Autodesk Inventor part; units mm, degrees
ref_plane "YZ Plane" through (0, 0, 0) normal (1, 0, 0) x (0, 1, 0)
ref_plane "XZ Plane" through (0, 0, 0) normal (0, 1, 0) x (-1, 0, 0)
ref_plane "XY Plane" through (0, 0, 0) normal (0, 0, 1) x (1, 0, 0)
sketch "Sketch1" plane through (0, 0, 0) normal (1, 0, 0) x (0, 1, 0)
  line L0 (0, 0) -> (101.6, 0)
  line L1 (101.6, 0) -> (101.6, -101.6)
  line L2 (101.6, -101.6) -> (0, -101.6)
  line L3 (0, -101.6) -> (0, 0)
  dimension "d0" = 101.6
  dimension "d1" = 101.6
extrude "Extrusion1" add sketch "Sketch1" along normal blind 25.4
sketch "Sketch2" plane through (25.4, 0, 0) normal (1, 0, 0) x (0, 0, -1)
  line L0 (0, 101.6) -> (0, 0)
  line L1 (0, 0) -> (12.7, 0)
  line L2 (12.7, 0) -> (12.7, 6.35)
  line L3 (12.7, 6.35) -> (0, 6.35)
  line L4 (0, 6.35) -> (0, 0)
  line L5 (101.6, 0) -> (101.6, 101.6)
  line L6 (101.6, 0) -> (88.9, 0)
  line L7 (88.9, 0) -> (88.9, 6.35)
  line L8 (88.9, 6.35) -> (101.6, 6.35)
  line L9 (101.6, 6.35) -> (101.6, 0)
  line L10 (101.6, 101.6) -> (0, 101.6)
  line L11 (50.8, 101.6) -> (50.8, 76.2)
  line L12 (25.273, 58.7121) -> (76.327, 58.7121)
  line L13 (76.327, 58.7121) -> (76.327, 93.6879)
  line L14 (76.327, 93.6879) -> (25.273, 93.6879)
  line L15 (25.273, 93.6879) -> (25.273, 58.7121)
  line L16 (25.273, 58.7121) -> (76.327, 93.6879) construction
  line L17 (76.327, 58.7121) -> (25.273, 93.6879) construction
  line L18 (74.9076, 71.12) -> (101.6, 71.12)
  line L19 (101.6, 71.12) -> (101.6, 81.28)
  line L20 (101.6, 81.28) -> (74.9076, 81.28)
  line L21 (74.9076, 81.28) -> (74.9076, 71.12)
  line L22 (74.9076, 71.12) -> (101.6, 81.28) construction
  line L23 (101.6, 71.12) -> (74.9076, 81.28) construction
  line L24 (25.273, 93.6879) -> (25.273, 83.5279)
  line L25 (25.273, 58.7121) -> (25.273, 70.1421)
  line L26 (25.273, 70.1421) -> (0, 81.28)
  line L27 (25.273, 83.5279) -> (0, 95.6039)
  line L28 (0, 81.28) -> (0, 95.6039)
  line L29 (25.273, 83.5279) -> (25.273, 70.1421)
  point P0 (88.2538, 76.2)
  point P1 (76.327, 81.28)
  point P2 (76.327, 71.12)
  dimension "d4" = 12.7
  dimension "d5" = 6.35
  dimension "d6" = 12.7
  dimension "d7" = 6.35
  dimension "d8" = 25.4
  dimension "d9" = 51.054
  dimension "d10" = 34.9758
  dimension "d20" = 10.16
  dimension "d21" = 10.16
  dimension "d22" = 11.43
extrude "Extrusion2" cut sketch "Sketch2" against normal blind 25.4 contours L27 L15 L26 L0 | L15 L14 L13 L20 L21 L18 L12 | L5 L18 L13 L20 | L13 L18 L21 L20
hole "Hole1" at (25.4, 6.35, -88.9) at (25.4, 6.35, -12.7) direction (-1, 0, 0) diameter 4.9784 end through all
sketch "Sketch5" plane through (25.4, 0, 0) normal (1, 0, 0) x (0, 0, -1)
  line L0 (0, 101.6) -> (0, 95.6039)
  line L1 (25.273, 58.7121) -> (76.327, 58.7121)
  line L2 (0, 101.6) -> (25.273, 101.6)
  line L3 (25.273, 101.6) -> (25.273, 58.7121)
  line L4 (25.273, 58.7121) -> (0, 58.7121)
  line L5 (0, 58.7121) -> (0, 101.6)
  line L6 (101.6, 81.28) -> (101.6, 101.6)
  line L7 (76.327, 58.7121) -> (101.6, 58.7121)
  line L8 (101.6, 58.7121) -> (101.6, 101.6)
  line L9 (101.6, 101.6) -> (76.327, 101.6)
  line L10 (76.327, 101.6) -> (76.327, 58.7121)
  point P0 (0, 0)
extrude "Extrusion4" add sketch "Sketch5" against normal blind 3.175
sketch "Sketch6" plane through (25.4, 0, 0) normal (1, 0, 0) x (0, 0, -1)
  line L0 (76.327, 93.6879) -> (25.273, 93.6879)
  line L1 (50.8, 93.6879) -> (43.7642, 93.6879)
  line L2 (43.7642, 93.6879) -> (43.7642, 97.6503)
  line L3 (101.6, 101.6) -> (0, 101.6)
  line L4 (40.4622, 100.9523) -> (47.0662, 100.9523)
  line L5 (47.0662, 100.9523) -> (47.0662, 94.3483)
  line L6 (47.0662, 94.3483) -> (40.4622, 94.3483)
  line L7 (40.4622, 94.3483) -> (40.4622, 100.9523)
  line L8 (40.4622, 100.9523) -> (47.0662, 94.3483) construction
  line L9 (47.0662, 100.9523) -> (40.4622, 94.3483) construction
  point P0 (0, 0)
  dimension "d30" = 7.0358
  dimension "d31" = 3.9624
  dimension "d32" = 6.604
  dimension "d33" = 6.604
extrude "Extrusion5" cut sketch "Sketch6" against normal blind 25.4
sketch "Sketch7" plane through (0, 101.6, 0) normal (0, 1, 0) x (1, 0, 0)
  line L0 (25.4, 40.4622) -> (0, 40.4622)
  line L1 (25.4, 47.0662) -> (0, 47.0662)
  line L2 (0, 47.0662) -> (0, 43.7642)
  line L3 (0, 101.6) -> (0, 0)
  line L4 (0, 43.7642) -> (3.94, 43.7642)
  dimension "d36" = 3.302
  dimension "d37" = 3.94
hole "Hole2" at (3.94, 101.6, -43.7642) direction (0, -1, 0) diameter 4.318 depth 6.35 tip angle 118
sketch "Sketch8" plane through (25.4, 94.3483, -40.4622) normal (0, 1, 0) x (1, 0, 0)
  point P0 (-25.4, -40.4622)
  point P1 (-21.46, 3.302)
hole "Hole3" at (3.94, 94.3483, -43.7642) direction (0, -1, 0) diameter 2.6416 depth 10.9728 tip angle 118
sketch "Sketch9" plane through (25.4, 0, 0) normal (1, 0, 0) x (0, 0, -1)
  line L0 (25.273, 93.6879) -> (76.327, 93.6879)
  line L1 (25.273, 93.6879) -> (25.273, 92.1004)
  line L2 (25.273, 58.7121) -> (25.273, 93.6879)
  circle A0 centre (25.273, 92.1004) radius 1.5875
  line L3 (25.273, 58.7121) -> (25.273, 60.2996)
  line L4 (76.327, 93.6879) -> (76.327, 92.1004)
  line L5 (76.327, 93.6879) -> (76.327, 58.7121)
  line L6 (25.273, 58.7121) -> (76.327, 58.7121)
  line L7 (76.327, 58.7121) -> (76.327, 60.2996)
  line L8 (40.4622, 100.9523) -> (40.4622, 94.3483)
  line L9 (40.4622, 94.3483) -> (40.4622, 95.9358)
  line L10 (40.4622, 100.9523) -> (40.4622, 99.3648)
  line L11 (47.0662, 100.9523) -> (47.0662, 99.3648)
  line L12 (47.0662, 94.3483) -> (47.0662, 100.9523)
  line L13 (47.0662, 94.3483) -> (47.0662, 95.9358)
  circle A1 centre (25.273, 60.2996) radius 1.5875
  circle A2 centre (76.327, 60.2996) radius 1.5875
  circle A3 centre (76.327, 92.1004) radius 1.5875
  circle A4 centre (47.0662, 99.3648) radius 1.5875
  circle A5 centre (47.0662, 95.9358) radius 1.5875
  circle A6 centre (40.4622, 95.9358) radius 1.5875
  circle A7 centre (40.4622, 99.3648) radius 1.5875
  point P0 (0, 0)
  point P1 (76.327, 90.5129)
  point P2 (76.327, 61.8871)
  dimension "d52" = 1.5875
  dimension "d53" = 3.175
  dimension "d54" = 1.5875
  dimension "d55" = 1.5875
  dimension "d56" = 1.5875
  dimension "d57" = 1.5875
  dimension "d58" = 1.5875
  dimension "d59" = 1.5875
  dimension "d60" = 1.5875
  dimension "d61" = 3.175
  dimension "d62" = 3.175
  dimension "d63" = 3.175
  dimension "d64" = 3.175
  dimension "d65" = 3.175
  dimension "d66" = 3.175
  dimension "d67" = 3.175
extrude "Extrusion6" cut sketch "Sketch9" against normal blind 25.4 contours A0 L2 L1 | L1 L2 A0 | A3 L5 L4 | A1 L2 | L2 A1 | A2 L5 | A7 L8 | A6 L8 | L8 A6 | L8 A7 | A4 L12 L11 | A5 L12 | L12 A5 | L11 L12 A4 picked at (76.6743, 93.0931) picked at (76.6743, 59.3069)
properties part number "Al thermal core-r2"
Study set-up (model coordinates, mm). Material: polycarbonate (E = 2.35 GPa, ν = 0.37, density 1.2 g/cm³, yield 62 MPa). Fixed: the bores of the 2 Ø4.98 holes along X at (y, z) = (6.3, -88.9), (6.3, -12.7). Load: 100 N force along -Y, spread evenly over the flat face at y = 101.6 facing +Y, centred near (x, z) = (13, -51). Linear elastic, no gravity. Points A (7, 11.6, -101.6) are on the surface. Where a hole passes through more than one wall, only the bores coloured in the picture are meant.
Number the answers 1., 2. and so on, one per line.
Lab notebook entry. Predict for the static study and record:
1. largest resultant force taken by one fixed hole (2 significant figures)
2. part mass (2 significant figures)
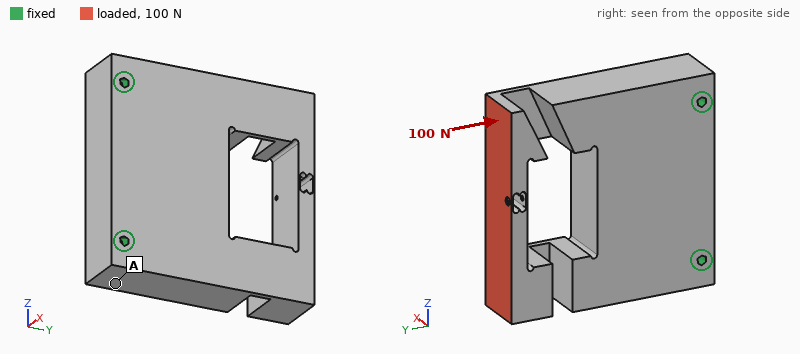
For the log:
1. 50 N
2. 240 g
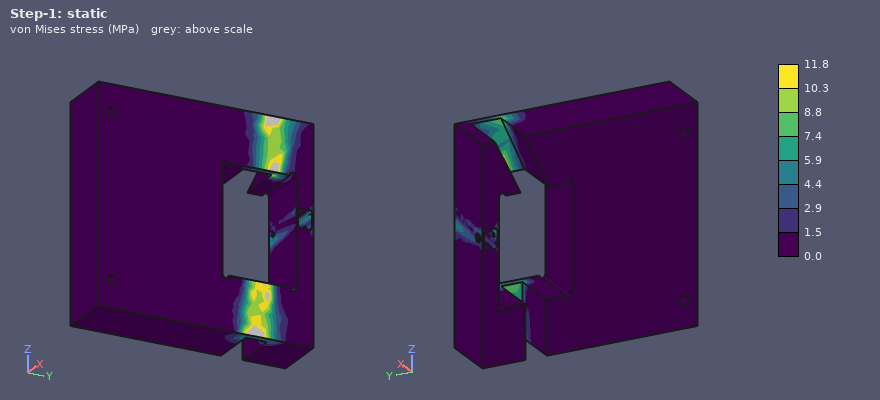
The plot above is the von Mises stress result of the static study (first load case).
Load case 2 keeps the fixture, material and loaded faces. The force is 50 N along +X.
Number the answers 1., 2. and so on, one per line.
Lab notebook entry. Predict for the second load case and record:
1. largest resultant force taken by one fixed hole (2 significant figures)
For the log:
1. 25 N
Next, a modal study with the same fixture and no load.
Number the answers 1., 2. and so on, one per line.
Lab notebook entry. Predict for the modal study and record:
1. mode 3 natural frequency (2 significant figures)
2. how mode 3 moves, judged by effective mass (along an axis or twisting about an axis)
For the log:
1. 700 Hz
2. along X
